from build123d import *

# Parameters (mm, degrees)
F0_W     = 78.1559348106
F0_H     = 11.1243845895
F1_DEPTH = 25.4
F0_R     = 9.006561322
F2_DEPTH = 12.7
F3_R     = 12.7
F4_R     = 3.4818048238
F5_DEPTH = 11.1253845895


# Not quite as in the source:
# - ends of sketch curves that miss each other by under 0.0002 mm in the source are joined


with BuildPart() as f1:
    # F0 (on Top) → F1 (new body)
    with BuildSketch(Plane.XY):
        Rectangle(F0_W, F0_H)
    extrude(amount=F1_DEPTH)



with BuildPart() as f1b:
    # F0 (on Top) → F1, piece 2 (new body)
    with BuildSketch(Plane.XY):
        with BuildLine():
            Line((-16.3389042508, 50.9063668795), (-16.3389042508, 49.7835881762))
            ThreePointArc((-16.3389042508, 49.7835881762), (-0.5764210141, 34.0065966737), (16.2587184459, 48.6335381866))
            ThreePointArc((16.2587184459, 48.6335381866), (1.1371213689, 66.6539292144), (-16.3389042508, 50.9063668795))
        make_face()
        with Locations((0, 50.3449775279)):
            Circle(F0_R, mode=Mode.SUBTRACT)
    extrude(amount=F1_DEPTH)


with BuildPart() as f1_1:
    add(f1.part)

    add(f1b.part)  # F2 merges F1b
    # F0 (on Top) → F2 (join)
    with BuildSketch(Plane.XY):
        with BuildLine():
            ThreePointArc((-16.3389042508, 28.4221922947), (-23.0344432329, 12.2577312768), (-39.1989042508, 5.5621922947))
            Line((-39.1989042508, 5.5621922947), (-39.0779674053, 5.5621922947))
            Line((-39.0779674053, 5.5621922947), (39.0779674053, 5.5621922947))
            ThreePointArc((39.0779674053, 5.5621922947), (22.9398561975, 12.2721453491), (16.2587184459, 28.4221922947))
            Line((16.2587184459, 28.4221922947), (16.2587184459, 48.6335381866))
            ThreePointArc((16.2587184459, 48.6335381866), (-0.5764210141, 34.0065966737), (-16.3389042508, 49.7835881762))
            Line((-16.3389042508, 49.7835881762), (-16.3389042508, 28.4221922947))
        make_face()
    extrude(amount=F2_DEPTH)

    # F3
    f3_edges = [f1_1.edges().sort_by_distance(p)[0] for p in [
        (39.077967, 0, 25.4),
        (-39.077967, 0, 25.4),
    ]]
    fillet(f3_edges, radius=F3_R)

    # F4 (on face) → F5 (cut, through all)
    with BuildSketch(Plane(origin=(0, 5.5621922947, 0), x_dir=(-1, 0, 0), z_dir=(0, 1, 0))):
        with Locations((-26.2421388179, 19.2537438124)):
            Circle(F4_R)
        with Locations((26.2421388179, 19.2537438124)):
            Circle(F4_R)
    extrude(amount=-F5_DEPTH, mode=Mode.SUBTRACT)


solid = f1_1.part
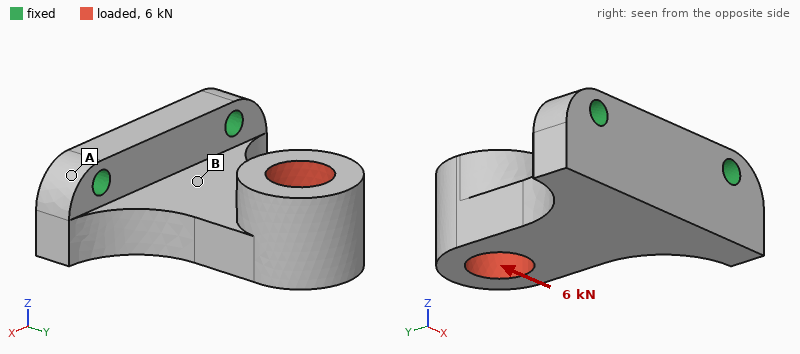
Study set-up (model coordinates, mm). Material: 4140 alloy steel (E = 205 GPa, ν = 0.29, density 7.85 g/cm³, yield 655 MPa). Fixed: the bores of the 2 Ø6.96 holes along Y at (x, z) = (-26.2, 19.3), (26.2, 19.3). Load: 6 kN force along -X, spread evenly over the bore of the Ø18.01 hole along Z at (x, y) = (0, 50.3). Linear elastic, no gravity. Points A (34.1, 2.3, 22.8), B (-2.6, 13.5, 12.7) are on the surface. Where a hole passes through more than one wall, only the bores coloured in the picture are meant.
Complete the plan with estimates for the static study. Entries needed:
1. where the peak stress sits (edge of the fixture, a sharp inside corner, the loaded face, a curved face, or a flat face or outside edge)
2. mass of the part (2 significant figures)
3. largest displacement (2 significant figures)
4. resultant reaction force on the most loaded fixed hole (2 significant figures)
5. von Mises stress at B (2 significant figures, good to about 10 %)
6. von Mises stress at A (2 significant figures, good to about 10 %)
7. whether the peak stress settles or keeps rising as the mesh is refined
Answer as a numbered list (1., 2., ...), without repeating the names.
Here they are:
1. edge of the fixture
2. 400 g
3. 81 µm
4. 6.5 kN
5. 44 MPa
6. 22 MPa
7. keeps rising
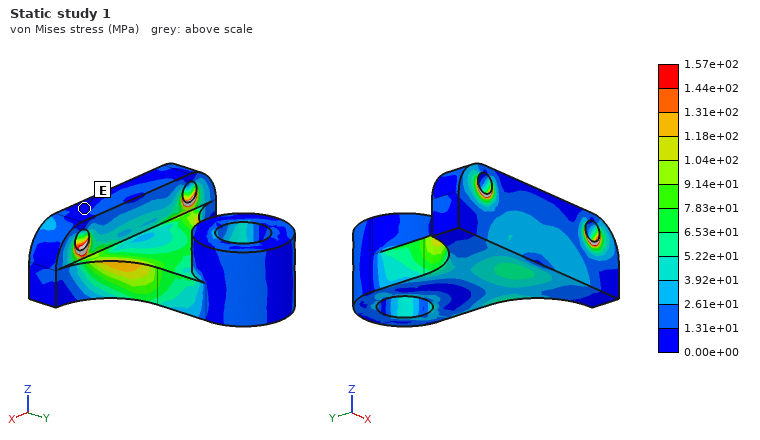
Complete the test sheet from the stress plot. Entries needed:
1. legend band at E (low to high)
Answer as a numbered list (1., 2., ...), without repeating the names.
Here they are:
1. 0.00e+00 to 1.31e+01 MPa
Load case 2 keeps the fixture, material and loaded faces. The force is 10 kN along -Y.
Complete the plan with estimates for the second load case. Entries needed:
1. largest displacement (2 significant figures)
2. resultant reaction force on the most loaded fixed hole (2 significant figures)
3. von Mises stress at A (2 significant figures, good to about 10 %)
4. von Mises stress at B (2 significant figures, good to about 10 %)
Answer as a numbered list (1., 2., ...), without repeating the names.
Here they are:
1. 87 µm
2. 5.1 kN
3. 14 MPa
4. 62 MPa
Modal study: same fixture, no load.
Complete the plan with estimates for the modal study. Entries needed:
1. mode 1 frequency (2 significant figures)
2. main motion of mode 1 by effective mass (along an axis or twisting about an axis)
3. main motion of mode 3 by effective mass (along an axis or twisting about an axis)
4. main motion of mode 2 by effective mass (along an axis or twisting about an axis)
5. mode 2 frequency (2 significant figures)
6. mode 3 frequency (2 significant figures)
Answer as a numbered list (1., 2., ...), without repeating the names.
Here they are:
1. 1800 Hz
2. along Z
3. along Y
4. along X
5. 4500 Hz
6. 7100 Hz
